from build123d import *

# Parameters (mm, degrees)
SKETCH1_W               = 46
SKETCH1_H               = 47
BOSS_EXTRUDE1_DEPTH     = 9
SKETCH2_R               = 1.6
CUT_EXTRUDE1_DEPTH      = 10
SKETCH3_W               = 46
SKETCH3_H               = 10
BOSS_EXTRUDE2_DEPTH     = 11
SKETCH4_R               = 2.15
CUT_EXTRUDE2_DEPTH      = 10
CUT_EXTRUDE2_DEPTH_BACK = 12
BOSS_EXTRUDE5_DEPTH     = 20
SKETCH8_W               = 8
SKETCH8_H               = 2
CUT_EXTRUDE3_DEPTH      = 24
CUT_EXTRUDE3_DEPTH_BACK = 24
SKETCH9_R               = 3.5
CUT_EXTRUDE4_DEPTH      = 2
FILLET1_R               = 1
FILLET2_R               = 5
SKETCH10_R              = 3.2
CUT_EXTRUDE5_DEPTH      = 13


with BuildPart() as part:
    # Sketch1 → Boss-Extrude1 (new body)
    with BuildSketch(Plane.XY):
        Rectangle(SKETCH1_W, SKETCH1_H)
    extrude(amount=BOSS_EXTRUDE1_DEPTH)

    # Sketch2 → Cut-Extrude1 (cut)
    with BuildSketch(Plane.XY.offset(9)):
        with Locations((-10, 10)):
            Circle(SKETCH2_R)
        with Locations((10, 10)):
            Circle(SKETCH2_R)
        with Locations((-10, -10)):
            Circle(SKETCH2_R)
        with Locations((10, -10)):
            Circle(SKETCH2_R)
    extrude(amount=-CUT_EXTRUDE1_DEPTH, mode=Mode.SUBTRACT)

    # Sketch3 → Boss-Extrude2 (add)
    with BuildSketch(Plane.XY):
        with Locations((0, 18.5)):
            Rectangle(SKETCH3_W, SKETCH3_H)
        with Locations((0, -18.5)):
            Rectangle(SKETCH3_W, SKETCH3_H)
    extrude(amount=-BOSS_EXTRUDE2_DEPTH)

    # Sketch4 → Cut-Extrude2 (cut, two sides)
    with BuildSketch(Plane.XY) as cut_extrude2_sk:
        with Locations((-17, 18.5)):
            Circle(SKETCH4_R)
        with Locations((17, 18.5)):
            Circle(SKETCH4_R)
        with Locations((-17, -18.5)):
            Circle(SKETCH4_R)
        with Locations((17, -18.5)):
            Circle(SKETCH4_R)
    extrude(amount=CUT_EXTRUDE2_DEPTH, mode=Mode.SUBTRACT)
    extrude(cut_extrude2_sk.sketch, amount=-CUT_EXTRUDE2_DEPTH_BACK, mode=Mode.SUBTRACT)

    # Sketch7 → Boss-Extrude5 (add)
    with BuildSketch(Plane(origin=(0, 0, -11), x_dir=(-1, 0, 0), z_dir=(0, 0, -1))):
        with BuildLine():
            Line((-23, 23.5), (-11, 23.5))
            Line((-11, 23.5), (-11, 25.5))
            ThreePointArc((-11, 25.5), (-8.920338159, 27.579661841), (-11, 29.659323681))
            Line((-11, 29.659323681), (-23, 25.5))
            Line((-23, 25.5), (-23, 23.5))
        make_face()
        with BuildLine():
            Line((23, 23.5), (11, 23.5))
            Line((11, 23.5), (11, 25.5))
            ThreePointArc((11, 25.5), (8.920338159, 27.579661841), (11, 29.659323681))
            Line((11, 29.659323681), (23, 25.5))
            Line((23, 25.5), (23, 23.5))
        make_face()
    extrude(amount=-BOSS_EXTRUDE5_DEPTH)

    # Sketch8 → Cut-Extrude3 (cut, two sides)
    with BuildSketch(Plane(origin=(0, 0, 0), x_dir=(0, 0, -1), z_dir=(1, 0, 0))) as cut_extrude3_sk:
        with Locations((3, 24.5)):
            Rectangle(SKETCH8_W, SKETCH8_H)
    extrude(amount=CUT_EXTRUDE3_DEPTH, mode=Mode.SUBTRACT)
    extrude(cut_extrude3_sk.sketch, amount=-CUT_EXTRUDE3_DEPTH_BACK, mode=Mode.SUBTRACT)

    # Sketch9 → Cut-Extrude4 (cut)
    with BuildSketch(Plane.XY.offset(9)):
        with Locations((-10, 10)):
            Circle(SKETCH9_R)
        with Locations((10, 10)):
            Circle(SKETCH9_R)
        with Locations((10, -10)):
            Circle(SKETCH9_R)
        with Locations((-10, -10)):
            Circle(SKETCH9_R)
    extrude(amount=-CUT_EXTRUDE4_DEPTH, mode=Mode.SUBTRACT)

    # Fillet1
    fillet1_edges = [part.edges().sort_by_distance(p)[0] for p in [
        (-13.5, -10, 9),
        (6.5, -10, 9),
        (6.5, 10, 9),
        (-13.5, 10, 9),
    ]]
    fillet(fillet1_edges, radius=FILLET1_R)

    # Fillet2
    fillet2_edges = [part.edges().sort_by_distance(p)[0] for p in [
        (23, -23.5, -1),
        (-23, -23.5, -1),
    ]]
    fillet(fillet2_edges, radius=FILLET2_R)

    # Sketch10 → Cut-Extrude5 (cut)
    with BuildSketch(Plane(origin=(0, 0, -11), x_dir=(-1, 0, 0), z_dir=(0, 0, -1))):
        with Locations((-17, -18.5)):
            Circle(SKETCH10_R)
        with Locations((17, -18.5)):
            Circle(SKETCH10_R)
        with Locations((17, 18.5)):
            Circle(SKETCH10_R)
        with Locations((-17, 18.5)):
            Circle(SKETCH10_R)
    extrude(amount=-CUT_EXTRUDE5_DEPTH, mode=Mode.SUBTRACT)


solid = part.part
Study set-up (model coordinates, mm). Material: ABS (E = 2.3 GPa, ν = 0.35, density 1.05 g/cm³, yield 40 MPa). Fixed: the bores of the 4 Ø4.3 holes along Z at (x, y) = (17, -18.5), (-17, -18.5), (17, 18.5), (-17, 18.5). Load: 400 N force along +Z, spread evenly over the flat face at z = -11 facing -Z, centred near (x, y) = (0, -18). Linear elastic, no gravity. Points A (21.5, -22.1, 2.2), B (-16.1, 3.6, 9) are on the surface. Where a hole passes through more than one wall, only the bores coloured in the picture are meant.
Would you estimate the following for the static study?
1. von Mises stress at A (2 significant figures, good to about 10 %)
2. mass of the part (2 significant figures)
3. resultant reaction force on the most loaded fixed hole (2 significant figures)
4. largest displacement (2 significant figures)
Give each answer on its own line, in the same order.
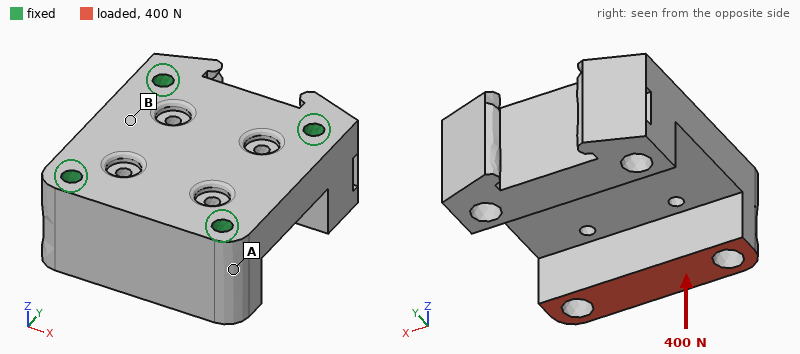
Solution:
1.3 MPa
30 g
210 N
24 µm
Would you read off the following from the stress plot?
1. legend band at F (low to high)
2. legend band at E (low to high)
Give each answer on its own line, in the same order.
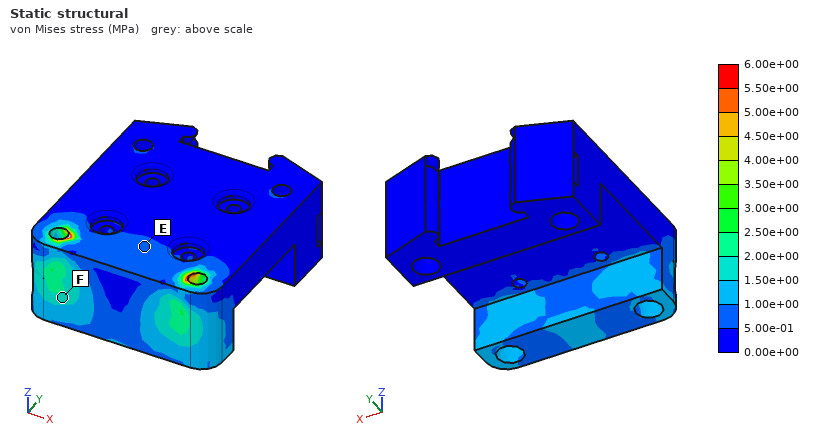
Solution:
1.50e+00 to 2.00e+00 MPa
5.00e-01 to 1.00e+00 MPa
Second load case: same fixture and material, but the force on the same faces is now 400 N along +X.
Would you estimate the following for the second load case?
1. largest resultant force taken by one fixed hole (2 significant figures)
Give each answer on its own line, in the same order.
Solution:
250 N
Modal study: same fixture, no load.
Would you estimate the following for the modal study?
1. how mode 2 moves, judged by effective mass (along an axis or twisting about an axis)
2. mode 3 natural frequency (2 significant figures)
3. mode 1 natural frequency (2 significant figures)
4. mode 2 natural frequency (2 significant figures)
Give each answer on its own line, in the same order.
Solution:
along Y
6800 Hz
4500 Hz
5600 Hz
